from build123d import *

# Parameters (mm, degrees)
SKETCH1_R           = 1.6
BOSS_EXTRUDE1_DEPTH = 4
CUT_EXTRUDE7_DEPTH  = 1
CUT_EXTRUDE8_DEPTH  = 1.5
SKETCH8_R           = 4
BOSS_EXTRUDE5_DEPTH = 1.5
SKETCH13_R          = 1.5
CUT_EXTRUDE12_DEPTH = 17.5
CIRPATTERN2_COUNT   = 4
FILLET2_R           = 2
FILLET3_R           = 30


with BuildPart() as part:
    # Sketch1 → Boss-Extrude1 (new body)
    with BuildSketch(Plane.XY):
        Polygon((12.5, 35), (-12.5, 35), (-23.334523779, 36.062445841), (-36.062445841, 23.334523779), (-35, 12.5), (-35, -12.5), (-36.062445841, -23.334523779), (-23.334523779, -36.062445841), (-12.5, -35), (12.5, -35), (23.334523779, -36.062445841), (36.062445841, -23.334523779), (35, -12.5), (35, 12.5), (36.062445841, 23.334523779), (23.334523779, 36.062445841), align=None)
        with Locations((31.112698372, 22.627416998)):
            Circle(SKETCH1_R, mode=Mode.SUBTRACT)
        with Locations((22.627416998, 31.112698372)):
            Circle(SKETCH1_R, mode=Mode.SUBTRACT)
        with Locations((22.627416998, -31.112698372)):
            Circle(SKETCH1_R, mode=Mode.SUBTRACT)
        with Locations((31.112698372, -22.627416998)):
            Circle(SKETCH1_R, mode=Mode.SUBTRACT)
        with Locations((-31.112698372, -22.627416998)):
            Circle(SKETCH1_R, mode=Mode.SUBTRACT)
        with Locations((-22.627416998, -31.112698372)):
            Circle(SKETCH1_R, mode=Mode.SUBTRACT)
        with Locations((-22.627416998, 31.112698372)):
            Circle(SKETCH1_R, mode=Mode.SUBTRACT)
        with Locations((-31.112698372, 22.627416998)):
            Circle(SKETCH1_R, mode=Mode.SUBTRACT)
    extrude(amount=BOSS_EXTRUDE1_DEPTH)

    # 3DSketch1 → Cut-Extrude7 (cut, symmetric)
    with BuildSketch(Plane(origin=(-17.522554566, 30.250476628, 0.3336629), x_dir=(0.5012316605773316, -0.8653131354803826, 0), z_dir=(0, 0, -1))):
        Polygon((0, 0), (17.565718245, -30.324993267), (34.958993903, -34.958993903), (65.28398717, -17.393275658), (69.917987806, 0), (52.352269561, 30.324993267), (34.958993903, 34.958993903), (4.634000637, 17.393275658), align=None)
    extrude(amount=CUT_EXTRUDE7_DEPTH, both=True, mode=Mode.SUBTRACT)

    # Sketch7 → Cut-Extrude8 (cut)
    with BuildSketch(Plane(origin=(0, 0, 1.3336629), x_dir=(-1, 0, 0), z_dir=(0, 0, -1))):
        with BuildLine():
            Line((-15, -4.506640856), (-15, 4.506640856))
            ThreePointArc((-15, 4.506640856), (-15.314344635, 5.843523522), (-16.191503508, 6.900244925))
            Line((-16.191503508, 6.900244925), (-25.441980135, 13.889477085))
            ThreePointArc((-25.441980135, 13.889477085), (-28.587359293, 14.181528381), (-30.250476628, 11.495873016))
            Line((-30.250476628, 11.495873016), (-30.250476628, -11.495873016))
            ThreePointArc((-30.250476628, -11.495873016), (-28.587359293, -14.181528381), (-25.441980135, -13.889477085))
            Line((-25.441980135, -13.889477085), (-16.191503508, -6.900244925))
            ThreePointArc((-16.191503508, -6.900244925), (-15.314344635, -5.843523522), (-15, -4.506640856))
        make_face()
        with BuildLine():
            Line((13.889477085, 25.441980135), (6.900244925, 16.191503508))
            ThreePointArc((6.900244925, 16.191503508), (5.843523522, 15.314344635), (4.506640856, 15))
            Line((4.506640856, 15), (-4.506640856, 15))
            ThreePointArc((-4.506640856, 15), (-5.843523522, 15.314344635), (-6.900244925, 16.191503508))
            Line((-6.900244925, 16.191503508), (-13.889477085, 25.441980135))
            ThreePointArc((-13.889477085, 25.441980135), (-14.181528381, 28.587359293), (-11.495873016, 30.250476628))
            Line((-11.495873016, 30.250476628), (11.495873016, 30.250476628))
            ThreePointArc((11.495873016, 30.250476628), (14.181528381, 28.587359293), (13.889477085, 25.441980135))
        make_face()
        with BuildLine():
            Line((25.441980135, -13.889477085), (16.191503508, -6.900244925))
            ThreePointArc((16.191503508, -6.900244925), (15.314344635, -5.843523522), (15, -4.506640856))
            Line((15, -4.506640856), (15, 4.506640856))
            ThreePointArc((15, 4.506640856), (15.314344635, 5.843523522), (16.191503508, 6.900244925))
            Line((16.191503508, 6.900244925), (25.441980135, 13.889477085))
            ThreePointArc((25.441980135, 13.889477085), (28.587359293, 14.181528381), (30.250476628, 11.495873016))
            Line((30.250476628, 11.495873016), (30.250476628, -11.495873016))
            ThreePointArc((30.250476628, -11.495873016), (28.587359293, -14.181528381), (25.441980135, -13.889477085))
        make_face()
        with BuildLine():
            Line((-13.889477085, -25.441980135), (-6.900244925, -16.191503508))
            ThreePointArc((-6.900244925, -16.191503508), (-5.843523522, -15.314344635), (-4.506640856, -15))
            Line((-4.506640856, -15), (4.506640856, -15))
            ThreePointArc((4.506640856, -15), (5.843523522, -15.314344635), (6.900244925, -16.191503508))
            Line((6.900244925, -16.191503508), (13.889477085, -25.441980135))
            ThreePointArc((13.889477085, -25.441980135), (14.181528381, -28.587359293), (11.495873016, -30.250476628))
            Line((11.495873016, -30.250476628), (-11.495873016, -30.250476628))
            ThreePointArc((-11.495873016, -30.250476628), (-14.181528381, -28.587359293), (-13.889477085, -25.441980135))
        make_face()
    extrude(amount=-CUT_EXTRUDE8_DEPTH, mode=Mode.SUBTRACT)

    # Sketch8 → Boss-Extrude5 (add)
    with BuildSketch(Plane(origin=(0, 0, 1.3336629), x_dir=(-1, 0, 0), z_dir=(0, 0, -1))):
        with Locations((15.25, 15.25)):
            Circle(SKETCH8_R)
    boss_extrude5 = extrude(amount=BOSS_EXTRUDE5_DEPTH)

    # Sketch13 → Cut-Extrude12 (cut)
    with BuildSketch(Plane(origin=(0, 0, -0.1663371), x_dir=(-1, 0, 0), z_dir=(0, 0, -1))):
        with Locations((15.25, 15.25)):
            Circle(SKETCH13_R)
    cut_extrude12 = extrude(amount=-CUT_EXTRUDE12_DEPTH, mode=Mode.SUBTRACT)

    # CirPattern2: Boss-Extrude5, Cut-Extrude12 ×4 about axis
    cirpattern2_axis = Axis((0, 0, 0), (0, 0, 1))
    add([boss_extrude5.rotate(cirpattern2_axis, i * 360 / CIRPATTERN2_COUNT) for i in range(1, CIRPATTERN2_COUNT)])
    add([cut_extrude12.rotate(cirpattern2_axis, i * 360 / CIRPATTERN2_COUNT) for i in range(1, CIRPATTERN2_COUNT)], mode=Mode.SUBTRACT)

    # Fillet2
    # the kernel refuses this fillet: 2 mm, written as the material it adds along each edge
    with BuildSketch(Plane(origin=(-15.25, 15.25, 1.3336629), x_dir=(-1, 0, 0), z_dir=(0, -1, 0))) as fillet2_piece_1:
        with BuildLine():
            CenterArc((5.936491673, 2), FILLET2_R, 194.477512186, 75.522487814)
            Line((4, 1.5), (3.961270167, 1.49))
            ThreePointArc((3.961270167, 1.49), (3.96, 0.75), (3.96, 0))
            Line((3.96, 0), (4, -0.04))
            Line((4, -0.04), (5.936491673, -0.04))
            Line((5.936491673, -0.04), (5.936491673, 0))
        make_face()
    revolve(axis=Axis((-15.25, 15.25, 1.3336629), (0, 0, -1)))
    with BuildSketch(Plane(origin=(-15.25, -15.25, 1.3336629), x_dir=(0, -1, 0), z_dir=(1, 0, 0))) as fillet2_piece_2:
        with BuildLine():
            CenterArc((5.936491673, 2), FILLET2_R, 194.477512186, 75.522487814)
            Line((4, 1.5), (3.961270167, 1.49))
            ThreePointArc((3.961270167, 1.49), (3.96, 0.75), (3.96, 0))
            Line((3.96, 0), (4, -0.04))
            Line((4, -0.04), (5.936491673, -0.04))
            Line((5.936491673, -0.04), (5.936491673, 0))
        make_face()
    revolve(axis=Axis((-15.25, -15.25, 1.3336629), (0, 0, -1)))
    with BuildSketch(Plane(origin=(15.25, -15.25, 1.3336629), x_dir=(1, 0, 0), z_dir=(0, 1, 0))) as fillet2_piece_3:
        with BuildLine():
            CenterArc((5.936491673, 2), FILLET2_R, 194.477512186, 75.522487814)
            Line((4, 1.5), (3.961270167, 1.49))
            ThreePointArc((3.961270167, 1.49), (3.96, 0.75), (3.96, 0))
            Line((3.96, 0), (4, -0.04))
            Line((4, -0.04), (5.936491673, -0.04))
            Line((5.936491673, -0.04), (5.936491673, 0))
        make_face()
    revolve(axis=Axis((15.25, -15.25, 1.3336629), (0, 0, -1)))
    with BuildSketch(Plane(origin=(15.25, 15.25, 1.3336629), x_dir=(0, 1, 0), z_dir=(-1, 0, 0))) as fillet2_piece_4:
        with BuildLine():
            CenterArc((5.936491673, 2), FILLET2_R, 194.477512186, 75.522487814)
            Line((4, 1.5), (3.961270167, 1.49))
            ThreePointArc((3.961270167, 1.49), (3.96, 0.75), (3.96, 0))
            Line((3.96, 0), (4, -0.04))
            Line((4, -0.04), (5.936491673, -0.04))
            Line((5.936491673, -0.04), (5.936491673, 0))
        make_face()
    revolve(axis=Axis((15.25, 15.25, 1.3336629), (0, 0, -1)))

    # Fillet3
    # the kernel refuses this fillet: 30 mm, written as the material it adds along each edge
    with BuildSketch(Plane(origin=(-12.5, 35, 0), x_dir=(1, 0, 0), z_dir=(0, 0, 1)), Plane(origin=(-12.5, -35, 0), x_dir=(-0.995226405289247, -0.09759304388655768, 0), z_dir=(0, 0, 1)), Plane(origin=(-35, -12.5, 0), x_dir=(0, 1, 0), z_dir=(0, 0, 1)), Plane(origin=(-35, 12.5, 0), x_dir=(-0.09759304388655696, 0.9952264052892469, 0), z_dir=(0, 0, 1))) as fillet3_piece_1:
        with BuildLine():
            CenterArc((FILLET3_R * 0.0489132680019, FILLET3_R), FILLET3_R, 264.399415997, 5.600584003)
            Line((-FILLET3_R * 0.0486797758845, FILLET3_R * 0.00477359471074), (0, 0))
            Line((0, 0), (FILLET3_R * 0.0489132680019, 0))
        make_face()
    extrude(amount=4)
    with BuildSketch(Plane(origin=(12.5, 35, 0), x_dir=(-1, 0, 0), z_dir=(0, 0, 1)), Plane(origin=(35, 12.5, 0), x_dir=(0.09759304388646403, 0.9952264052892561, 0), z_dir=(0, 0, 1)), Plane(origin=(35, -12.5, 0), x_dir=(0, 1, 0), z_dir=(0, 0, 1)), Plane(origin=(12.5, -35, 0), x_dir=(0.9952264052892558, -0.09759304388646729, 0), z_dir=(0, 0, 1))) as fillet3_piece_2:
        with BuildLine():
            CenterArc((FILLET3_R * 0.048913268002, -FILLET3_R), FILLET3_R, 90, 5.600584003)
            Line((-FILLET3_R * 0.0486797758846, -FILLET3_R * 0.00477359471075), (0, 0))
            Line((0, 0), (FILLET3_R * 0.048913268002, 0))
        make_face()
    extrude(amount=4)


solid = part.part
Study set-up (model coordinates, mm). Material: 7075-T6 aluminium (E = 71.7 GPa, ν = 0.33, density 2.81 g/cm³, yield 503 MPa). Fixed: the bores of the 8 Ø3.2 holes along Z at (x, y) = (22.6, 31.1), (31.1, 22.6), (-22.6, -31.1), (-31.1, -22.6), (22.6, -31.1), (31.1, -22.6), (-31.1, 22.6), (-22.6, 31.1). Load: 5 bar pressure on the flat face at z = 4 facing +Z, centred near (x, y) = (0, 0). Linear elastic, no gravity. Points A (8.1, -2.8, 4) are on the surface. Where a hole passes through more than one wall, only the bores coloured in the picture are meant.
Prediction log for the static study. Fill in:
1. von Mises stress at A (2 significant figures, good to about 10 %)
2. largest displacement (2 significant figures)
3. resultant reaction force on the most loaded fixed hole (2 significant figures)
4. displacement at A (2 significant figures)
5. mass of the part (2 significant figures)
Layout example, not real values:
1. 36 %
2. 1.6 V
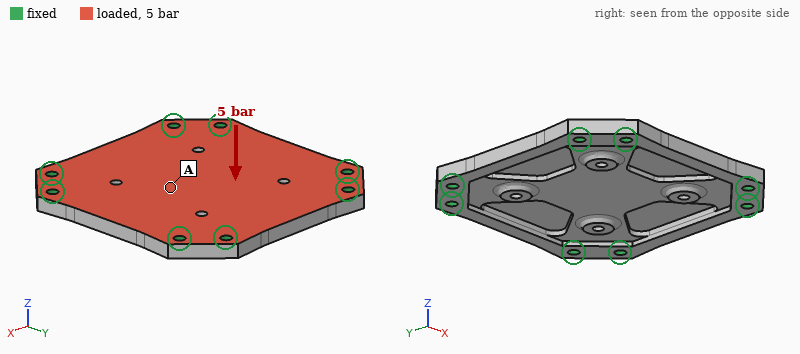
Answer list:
1. 51 MPa
2. 0.18 mm
3. 360 N
4. 0.16 mm
5. 35 g
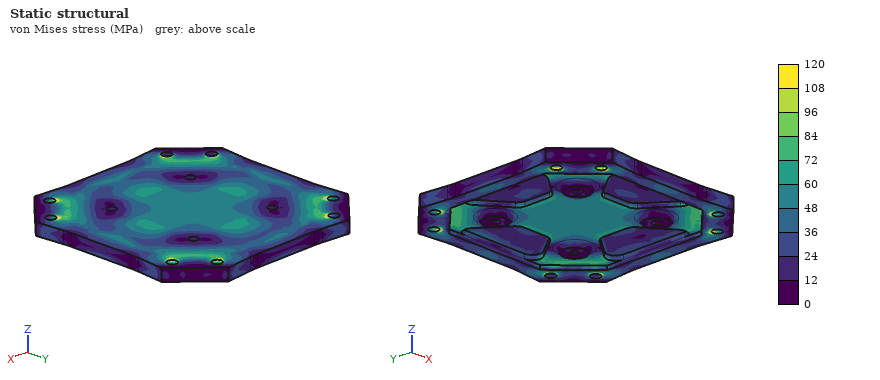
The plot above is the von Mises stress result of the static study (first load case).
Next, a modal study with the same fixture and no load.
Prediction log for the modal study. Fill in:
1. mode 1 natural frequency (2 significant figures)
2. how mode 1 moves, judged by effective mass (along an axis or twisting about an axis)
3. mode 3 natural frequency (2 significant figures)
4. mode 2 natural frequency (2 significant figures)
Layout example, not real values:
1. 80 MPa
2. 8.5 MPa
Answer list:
1. 4000 Hz
2. along Z
3. 8300 Hz
4. 8300 Hz
